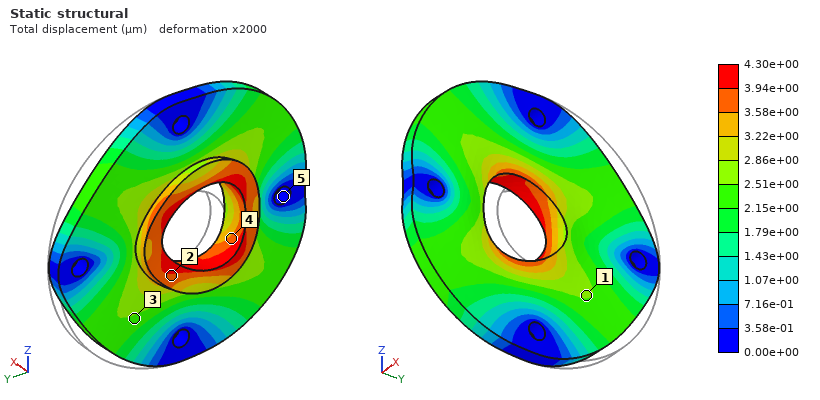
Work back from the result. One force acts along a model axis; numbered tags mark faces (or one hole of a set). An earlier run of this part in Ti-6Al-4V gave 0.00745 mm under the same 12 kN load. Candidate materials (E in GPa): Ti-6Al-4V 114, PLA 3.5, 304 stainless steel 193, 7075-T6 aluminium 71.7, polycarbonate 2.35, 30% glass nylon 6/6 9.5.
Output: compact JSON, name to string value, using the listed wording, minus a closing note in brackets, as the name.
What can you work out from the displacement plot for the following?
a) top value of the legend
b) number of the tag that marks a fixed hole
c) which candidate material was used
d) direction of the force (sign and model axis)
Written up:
{"top value of the legend": "4.30e+00 µm", "number of the tag that marks a fixed hole": "5", "which candidate material was used": "304 stainless steel", "direction of the force": "-Y"}
